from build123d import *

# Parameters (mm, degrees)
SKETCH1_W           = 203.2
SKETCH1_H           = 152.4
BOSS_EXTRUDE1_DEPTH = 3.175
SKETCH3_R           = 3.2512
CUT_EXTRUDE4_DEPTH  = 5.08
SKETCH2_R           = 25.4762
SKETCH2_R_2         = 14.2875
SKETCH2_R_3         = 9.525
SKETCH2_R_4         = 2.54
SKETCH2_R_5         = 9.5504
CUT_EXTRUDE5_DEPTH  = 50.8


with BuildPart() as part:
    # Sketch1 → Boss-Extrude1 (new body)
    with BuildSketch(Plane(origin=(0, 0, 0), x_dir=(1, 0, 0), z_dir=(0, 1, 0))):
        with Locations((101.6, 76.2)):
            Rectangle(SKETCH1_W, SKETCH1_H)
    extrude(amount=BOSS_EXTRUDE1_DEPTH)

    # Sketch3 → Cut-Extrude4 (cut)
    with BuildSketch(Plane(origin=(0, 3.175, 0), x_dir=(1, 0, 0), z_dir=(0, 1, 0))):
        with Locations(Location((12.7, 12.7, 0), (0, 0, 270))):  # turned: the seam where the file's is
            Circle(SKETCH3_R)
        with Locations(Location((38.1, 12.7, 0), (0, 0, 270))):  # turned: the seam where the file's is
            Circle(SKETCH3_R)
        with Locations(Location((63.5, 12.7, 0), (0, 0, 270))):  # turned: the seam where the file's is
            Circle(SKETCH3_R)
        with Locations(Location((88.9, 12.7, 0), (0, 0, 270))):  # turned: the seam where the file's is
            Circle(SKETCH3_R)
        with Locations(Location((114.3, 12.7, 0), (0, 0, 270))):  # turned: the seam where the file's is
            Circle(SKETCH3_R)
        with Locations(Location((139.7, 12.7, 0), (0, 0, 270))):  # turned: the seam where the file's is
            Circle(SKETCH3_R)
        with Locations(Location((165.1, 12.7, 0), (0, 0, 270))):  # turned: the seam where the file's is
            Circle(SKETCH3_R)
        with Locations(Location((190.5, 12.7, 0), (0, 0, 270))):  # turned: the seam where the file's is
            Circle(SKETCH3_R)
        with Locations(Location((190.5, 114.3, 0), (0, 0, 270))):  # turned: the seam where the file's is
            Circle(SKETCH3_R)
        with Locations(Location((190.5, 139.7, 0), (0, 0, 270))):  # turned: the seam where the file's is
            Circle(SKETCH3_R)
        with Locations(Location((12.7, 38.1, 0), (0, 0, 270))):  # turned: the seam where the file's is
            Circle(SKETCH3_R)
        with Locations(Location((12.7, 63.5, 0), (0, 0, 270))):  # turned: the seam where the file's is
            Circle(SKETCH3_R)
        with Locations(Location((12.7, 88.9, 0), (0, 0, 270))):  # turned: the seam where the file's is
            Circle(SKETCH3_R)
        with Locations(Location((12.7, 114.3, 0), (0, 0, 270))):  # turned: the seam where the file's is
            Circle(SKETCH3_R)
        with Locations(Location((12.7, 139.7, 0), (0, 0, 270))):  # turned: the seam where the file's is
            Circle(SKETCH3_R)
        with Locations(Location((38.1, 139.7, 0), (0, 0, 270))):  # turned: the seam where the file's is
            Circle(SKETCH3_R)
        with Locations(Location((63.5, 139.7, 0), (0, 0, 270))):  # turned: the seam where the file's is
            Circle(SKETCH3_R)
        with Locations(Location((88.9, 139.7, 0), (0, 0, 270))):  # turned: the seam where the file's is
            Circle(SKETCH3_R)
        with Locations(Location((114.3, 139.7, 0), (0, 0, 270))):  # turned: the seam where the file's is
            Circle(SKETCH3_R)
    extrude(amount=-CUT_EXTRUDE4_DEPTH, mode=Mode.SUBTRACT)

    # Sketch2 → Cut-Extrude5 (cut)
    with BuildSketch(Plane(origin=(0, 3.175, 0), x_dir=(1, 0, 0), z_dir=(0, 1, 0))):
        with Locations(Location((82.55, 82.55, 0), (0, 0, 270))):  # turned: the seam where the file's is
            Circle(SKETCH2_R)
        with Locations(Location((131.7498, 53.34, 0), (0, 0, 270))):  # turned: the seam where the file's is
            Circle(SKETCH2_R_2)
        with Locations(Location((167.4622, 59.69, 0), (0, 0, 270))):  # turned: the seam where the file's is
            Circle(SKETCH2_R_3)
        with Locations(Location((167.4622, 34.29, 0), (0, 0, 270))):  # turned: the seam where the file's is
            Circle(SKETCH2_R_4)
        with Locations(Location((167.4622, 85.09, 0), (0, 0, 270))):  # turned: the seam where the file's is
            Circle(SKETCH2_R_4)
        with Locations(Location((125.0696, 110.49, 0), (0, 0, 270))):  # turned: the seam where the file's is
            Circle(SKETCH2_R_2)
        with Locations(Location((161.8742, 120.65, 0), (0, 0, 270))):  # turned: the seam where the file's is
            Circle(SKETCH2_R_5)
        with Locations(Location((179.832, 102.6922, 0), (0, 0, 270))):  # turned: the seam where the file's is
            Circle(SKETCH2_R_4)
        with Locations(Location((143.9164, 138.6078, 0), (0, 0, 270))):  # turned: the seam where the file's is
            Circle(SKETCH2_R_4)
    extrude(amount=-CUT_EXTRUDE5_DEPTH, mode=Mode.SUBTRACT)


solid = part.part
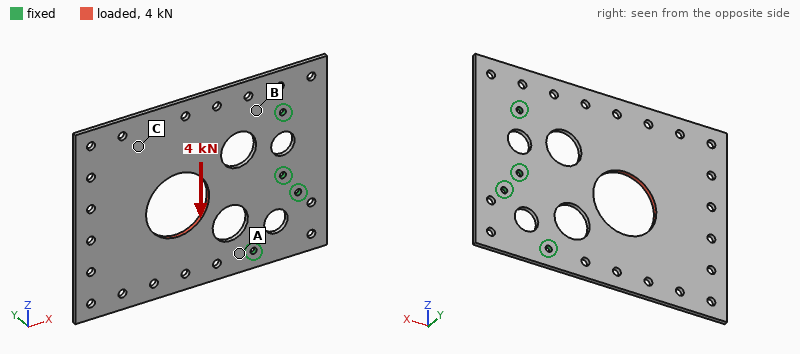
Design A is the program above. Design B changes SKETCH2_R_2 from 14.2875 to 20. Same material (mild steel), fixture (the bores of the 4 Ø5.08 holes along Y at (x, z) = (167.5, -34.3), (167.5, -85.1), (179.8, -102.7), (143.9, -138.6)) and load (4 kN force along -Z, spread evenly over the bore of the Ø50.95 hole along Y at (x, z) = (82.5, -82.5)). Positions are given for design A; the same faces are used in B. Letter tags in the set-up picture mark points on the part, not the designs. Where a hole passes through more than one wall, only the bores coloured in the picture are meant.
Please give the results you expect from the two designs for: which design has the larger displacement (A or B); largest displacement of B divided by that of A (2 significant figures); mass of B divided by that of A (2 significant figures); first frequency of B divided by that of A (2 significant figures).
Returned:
B
1.4
0.95
0.90
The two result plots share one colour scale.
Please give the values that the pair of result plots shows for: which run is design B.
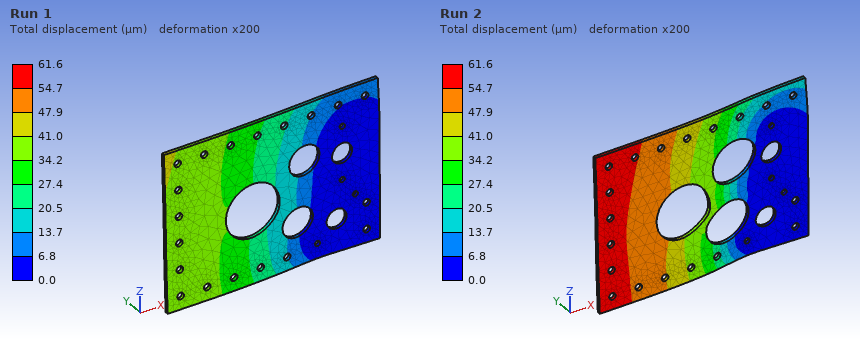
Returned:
Run 2
